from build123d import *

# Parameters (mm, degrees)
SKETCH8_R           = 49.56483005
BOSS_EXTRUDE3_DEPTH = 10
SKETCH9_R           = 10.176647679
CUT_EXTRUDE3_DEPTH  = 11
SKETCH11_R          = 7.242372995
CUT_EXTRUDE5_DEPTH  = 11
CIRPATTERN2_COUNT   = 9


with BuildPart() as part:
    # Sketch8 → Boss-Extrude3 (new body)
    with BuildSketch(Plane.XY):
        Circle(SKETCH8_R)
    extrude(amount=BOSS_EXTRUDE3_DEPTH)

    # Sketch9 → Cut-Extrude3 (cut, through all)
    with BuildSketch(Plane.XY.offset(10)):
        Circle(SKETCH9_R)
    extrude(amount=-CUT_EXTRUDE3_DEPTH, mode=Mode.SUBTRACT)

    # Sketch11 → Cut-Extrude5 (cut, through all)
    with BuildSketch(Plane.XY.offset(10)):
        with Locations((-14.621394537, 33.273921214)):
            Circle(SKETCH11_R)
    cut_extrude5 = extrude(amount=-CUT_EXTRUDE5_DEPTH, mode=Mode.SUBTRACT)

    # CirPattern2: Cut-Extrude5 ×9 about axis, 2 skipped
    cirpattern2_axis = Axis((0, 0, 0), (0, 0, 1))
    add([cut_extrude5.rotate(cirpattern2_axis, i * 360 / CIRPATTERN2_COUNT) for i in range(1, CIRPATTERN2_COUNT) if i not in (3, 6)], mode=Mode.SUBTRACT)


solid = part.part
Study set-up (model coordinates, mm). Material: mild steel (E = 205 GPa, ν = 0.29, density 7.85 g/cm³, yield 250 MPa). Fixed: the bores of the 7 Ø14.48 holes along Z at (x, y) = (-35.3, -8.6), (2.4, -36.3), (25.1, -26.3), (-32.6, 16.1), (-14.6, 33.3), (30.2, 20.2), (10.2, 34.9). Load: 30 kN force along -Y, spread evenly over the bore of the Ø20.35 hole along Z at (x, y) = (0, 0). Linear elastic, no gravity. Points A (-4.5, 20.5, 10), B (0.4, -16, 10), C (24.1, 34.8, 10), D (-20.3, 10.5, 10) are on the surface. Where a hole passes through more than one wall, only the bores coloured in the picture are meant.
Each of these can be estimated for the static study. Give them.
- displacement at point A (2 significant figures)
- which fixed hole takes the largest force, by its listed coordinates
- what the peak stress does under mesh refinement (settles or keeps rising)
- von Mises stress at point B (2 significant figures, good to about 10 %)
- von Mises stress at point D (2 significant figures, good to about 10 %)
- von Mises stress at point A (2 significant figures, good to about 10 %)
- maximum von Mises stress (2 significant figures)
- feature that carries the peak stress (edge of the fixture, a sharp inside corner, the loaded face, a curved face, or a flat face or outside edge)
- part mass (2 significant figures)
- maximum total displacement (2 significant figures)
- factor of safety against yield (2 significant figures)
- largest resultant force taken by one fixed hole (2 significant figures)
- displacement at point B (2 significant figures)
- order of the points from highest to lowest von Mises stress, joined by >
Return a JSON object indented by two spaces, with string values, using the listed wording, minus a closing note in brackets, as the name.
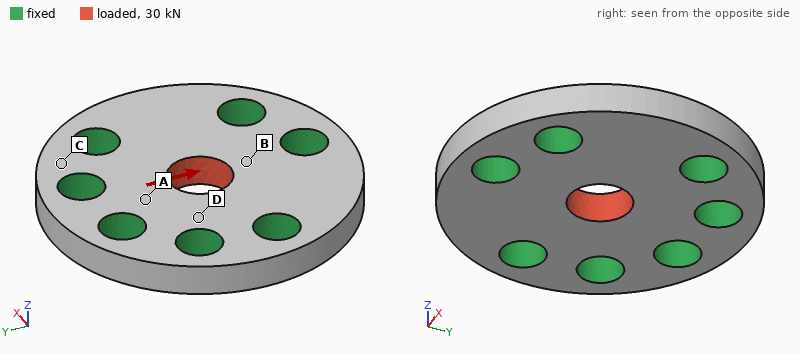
{
  "displacement at point A": "1.6 µm",
  "which fixed hole takes the largest force, by its listed coordinates": "(2.4, -36.3)",
  "what the peak stress does under mesh refinement": "settles",
  "von Mises stress at point B": "46 MPa",
  "von Mises stress at point D": "22 MPa",
  "von Mises stress at point A": "34 MPa",
  "maximum von Mises stress": "82 MPa",
  "feature that carries the peak stress": "the loaded face",
  "part mass": "490 g",
  "maximum total displacement": "4.7 µm",
  "factor of safety against yield": "3.0",
  "largest resultant force taken by one fixed hole": "7.7 kN",
  "displacement at point B": "2.9 µm",
  "order of the points from highest to lowest von Mises stress, joined by >": "B > A > D > C"
}
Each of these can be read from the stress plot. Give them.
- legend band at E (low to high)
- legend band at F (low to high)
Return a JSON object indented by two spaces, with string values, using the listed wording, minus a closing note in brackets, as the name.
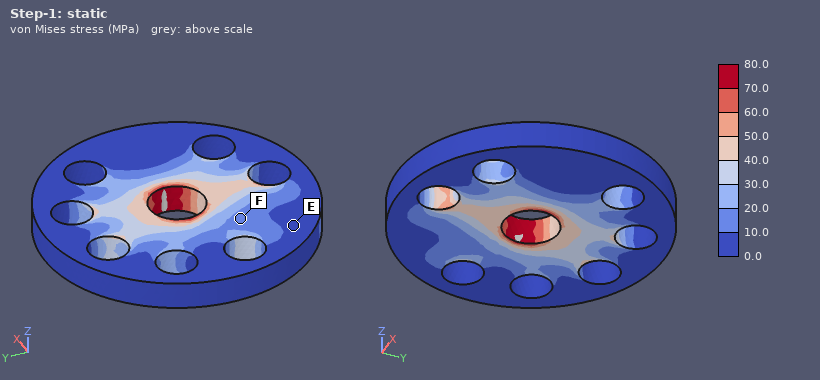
{
  "legend band at E": "0.0 to 10.0 MPa",
  "legend band at F": "10.0 to 20.0 MPa"
}
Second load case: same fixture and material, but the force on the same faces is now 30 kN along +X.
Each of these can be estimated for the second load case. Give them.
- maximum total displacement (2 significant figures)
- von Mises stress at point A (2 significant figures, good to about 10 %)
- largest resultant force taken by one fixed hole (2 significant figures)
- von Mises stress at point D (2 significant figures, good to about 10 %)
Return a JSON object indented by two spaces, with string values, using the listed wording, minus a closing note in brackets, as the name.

{
  "maximum total displacement": "5.1 µm",
  "von Mises stress at point A": "21 MPa",
  "largest resultant force taken by one fixed hole": "7.4 kN",
  "von Mises stress at point D": "34 MPa"
}
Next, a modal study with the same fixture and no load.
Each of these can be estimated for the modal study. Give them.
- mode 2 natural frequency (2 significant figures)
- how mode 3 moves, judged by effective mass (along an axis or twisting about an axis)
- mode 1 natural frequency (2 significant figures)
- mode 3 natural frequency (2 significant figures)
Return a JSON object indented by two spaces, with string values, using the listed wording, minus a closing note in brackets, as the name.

{
  "mode 2 natural frequency": "19 kHz",
  "how mode 3 moves, judged by effective mass": "along Z",
  "mode 1 natural frequency": "19 kHz",
  "mode 3 natural frequency": "22 kHz"
}
